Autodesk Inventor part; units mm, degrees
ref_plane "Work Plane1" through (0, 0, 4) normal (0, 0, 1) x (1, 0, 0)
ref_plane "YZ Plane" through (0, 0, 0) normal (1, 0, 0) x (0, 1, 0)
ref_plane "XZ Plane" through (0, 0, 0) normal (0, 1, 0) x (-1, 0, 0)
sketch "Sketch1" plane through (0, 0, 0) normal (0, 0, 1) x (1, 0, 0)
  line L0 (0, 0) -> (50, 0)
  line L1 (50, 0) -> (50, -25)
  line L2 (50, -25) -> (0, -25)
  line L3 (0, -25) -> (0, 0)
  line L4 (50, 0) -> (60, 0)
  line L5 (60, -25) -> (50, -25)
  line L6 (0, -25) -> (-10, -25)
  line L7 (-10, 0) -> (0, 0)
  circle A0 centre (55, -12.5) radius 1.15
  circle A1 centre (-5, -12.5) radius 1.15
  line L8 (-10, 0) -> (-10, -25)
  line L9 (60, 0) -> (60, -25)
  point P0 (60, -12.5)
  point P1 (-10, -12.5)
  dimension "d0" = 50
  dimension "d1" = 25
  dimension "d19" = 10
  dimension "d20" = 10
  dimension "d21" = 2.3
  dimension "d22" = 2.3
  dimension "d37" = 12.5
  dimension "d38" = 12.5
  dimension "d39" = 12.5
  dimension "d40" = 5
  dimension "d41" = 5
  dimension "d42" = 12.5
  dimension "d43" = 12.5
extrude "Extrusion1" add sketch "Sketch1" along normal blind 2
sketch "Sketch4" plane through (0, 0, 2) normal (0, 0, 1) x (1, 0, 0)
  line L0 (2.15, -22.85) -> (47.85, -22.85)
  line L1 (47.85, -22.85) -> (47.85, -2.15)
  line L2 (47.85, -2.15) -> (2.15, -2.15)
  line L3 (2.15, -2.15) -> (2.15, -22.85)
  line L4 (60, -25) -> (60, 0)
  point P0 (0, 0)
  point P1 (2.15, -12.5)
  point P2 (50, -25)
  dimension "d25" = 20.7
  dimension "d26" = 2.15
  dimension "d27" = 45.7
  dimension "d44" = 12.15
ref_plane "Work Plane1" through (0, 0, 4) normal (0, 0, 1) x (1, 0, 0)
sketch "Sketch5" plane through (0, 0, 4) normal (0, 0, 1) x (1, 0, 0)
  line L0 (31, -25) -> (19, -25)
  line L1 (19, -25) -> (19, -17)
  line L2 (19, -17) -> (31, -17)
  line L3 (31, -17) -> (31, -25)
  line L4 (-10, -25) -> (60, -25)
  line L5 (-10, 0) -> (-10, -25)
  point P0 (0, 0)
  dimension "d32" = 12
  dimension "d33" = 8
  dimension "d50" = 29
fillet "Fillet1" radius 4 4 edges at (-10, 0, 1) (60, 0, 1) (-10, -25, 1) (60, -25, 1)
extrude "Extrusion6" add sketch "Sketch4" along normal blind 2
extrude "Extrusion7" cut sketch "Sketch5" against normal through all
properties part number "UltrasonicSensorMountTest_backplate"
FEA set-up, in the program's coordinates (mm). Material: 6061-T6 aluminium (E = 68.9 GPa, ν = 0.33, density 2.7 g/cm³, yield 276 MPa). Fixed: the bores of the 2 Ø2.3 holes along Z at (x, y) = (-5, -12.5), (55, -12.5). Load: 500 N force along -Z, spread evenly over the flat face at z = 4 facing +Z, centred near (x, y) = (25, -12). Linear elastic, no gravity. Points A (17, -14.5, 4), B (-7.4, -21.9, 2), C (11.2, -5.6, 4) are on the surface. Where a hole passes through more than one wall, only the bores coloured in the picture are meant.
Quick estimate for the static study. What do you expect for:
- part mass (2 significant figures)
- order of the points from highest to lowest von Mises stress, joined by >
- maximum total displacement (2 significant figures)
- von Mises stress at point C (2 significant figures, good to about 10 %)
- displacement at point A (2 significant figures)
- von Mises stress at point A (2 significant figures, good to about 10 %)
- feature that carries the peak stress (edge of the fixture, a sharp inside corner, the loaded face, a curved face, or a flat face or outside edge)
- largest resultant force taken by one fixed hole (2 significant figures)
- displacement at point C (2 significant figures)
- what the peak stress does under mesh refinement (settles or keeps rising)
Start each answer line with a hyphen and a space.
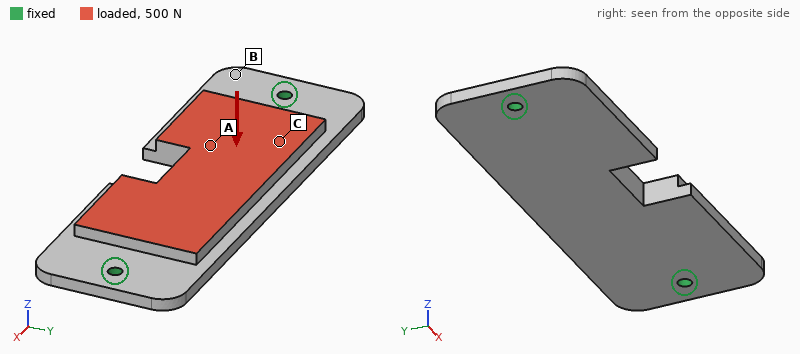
- 14 g
- A > C > B
- 0.14 mm
- 38 MPa
- 0.12 mm
- 60 MPa
- edge of the fixture
- 560 N
- 0.098 mm
- keeps rising
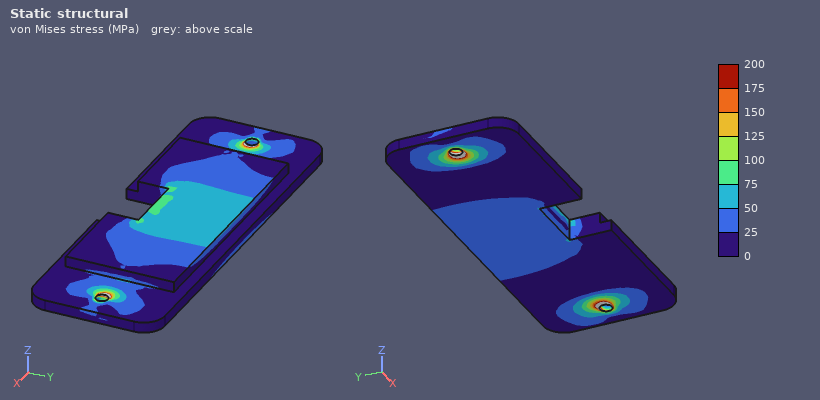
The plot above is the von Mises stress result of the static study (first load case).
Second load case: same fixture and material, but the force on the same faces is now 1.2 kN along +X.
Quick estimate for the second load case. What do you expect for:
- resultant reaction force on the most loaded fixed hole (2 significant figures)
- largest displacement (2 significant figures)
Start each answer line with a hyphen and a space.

- 600 N
- 6.7 µm
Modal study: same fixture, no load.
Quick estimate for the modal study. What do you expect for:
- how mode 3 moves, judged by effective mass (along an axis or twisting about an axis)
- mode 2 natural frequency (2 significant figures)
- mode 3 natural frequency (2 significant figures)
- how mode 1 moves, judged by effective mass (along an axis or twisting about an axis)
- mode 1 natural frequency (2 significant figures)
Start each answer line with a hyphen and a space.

- twisting about Y
- 4200 Hz
- 8600 Hz
- along Z
- 3400 Hz
